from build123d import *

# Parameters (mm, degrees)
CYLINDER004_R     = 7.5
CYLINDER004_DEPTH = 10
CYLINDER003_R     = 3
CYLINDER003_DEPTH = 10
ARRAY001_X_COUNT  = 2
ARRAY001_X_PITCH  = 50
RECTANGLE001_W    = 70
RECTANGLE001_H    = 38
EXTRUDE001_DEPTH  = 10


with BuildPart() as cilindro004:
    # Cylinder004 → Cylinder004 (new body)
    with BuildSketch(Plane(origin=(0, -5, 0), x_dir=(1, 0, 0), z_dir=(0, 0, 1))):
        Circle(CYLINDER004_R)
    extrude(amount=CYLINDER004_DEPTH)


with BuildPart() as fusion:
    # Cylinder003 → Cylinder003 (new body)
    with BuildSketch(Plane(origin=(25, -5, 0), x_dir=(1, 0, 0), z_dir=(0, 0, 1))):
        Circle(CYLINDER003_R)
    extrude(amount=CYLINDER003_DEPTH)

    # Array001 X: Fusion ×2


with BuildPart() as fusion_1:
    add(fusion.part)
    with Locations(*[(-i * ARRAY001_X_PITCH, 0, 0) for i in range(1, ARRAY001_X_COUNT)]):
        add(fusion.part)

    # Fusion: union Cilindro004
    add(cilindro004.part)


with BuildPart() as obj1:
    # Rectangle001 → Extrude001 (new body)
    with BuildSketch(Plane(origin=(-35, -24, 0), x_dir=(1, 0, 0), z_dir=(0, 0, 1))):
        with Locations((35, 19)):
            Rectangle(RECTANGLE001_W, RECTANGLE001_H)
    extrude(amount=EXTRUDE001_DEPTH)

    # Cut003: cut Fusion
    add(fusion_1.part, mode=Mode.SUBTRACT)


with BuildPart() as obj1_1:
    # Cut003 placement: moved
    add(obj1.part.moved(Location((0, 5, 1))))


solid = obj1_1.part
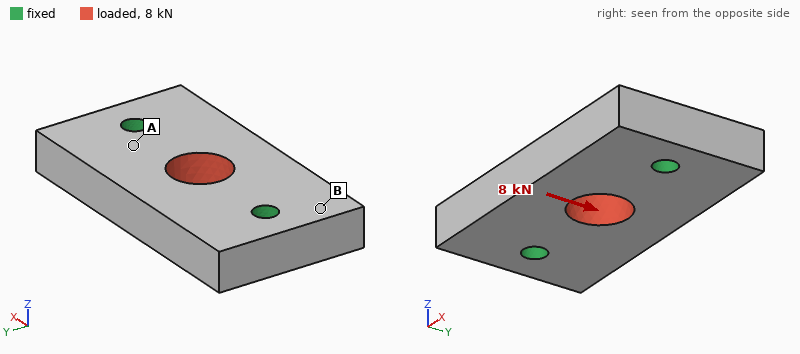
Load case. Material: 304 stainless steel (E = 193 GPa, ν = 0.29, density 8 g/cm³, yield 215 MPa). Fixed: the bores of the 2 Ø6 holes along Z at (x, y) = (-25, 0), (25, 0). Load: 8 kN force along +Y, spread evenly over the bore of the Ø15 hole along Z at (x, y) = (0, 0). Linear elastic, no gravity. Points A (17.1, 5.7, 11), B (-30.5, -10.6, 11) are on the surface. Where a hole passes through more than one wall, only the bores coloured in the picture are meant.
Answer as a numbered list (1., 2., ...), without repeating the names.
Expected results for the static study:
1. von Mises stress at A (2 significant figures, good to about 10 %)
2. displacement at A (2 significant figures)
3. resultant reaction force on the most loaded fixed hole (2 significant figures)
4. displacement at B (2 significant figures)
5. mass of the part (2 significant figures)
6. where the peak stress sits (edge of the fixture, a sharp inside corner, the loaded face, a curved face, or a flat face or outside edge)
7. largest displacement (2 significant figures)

1. 25 MPa
2. 2.1 µm
3. 4.0 kN
4. 0.98 µm
5. 190 g
6. edge of the fixture
7. 5.6 µm
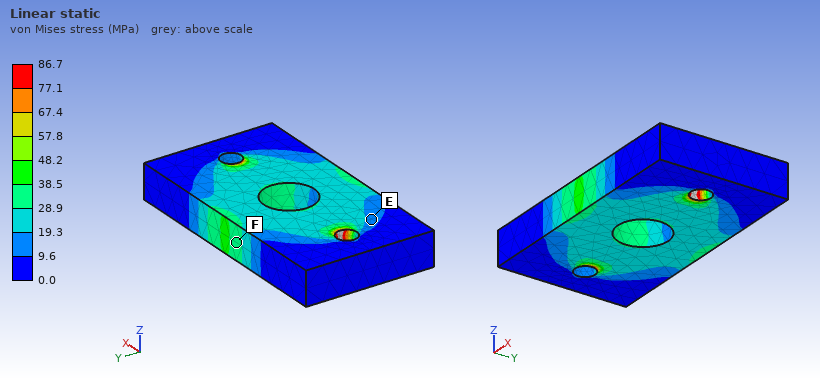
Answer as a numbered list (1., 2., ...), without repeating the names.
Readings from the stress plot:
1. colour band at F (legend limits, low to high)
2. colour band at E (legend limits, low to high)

1. 28.9 to 38.5 MPa
2. 9.6 to 19.3 MPa
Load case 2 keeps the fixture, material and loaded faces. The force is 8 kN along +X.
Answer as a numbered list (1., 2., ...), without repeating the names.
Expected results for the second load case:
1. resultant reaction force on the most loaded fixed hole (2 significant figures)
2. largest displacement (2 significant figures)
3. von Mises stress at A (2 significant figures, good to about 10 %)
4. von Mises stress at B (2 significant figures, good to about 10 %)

1. 4.0 kN
2. 2.4 µm
3. 17 MPa
4. 4.1 MPa
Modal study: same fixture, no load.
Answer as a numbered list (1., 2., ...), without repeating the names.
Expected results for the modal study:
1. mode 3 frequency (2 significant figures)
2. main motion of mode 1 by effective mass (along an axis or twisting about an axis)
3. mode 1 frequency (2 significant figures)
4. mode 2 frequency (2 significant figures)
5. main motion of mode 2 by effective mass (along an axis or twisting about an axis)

1. 19 kHz
2. twisting about X
3. 12 kHz
4. 13 kHz
5. along Z
